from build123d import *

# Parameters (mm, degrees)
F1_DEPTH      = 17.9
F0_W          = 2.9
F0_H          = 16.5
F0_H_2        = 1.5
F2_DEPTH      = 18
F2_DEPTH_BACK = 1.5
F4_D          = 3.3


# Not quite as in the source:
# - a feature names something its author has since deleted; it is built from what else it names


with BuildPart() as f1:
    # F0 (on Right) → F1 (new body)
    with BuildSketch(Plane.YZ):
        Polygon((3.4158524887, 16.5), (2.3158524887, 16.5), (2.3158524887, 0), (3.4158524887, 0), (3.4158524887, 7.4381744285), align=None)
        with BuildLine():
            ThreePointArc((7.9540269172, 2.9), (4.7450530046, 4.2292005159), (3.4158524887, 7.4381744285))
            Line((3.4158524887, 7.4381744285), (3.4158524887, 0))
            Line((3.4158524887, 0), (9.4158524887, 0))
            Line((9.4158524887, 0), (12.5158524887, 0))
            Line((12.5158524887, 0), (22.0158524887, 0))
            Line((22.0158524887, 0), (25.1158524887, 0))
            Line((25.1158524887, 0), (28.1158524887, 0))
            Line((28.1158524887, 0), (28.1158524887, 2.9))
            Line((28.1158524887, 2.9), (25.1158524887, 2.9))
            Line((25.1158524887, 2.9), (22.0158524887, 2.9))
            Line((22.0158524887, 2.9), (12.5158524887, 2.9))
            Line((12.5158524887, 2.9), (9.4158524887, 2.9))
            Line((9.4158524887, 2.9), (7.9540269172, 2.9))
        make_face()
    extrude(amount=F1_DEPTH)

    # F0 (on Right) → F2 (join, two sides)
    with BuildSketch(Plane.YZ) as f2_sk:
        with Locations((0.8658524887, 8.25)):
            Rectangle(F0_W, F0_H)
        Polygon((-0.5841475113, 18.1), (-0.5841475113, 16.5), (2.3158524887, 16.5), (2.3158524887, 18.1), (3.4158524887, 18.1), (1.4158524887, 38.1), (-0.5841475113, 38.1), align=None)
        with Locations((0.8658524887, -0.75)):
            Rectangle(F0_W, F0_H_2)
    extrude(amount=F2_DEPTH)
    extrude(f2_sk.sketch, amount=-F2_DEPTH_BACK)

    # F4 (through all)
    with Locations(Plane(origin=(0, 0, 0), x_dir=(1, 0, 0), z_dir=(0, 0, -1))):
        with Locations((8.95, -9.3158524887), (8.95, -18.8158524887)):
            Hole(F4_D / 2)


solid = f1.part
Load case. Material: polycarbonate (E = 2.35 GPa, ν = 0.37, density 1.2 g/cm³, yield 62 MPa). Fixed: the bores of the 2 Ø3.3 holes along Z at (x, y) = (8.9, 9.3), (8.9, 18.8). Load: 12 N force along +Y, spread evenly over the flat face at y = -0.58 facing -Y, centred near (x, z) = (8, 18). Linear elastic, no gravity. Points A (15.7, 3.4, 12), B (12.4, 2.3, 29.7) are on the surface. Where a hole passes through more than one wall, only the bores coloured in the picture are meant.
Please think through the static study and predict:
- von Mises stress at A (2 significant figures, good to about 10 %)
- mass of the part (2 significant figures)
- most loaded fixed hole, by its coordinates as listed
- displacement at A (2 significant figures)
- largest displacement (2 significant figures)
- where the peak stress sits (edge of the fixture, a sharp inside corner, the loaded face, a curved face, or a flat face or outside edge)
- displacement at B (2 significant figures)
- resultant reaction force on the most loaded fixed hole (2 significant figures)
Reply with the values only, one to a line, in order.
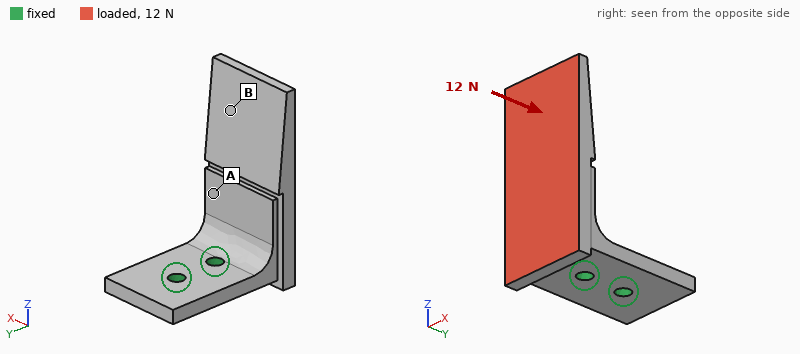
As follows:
2.0 MPa
4.7 g
(8.9, 9.3)
0.12 mm
0.62 mm
a curved face
0.44 mm
13 N
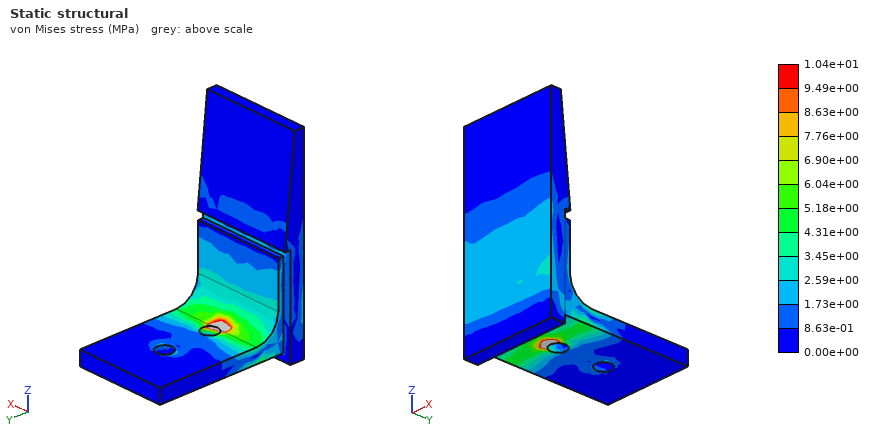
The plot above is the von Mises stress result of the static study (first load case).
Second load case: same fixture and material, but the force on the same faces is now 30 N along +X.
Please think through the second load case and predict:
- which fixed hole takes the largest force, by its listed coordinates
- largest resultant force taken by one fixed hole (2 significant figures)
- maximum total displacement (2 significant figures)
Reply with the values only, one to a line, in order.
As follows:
(8.9, 9.3)
49 N
0.60 mm
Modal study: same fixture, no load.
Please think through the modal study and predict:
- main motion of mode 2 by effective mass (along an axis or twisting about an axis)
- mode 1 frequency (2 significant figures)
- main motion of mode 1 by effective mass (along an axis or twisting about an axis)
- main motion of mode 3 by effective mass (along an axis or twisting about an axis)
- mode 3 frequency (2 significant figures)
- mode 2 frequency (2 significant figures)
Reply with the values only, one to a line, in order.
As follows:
along X
540 Hz
along Y
along Z
2400 Hz
810 Hz
